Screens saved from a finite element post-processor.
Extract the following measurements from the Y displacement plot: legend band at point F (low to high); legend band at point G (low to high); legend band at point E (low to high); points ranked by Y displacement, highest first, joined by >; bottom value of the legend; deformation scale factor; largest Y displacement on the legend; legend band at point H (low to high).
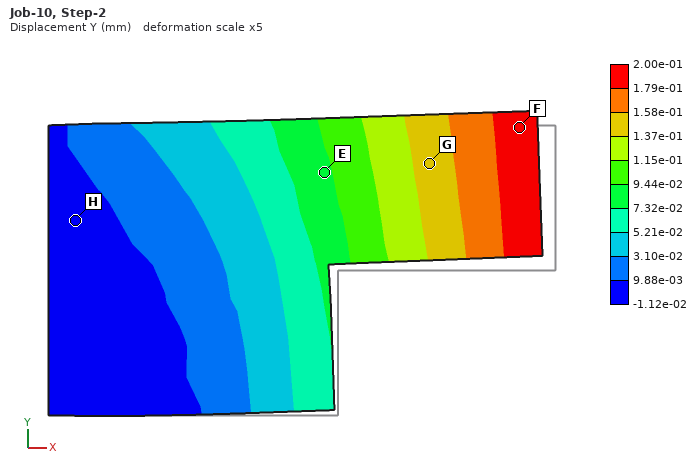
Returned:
1.79e-01 to 2.00e-01 mm
1.37e-01 to 1.58e-01 mm
7.32e-02 to 9.44e-02 mm
F > G > E > H
-1.12e-02 mm
5
2.00e-01 mm
-1.12e-02 to 9.88e-03 mm
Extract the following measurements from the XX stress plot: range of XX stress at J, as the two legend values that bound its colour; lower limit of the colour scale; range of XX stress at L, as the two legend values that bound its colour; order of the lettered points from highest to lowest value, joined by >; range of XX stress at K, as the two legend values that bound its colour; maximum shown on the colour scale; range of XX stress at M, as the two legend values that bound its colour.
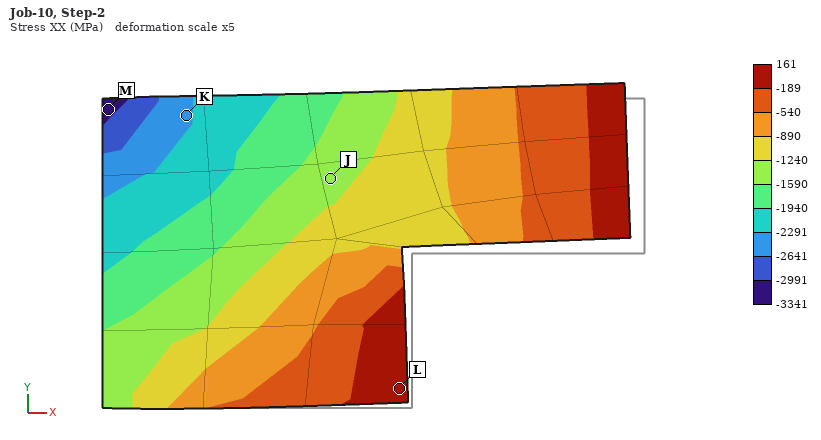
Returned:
-1590 to -1240 MPa
-3341 MPa
-189 to 161 MPa
L > J > K > M
-2641 to -2291 MPa
161 MPa
-3341 to -2991 MPa
